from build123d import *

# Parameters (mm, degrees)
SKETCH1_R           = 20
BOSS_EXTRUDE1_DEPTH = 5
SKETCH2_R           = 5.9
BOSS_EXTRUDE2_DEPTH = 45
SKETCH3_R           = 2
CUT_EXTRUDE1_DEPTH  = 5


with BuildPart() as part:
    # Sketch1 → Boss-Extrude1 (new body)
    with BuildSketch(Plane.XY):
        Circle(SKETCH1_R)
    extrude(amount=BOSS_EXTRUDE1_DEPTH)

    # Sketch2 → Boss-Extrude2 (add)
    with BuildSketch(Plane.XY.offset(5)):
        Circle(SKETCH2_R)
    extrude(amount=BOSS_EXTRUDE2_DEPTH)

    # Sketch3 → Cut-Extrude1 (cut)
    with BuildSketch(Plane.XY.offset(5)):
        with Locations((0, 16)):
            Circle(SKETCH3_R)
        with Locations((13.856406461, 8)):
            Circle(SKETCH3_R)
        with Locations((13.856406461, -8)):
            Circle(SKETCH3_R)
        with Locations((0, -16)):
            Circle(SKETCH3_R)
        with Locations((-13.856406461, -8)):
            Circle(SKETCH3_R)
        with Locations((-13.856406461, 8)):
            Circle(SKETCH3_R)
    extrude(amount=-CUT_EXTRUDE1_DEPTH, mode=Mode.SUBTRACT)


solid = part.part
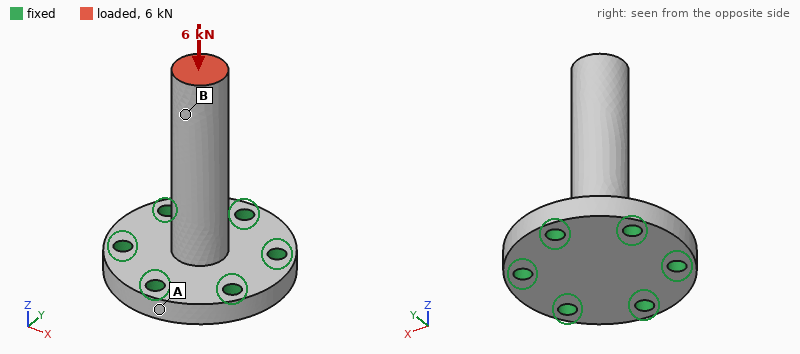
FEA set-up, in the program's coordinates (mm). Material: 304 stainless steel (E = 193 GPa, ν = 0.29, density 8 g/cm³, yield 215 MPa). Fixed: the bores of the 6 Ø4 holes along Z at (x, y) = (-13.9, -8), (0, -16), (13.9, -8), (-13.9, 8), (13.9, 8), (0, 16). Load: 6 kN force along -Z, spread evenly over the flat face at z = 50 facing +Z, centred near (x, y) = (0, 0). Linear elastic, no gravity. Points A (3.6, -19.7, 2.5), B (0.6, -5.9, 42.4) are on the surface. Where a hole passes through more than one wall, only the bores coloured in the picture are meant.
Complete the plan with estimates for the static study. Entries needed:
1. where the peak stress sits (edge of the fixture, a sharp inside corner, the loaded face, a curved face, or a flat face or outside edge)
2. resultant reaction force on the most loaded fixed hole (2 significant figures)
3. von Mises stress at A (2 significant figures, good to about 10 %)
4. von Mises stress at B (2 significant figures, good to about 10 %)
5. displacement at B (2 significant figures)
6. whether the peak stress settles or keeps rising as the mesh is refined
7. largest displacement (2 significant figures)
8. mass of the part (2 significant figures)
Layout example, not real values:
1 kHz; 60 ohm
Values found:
edge of the fixture; 1.0 kN; 22 MPa; 55 MPa; 20 µm; keeps rising; 22 µm; 87 g
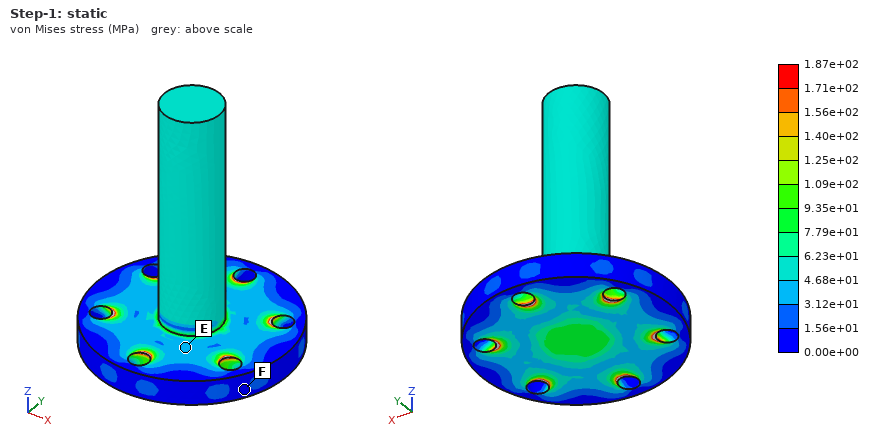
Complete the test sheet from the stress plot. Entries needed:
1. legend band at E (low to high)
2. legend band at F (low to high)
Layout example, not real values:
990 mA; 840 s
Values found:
3.12e+01 to 4.68e+01 MPa; 0.00e+00 to 1.56e+01 MPa
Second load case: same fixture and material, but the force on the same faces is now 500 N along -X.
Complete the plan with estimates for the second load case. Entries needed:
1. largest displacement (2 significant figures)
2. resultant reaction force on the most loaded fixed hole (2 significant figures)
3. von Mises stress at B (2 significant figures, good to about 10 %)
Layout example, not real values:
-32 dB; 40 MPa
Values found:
0.12 mm; 570 N; 9.9 MPa
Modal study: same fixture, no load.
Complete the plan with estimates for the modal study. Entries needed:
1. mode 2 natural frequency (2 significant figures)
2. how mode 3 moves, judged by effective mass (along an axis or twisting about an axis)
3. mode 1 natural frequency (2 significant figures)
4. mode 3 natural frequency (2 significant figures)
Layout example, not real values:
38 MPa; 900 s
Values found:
3100 Hz; along Z; 3100 Hz; 16 kHz
